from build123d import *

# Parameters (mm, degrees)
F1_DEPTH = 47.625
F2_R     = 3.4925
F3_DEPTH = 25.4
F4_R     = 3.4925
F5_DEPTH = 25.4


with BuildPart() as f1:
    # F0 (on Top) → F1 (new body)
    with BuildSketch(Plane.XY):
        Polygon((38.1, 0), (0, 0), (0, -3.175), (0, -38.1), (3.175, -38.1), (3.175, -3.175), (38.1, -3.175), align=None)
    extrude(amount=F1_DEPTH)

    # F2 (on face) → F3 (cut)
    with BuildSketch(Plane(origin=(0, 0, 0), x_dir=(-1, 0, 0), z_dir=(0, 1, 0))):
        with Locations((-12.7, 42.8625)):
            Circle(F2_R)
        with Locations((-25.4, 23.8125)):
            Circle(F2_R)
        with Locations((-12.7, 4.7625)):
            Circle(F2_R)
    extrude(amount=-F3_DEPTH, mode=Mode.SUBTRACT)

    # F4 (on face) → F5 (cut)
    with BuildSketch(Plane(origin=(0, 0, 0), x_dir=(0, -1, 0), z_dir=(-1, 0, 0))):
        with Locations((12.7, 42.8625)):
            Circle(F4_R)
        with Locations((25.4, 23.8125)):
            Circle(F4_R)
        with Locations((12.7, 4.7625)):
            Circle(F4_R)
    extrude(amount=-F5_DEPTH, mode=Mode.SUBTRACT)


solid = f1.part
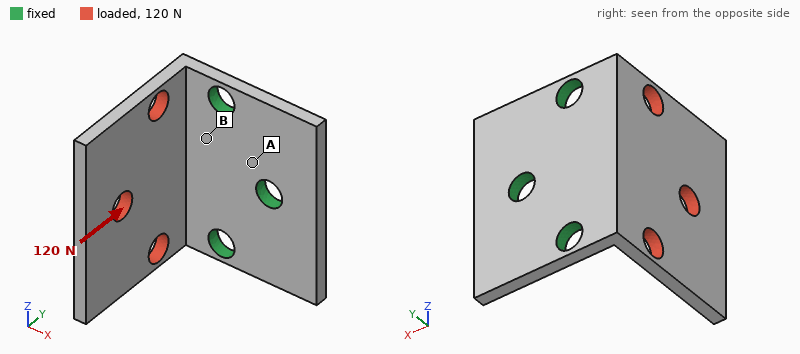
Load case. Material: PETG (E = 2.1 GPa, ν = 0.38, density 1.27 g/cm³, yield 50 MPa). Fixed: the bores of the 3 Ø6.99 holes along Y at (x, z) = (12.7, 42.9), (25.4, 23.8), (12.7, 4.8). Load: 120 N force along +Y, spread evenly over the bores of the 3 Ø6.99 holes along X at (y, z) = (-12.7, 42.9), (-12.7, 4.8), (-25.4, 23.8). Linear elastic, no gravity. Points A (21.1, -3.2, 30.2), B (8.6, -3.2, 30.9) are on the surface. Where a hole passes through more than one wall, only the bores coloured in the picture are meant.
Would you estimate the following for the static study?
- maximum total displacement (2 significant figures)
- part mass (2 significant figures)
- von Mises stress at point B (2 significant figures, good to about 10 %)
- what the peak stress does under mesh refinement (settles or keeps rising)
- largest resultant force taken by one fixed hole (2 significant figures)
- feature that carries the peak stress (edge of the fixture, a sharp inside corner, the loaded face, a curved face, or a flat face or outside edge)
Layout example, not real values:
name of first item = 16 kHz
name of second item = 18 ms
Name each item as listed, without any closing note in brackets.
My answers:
maximum total displacement = 0.71 mm
part mass = 13 g
von Mises stress at point B = 4.3 MPa
what the peak stress does under mesh refinement = keeps rising
largest resultant force taken by one fixed hole = 65 N
feature that carries the peak stress = edge of the fixture
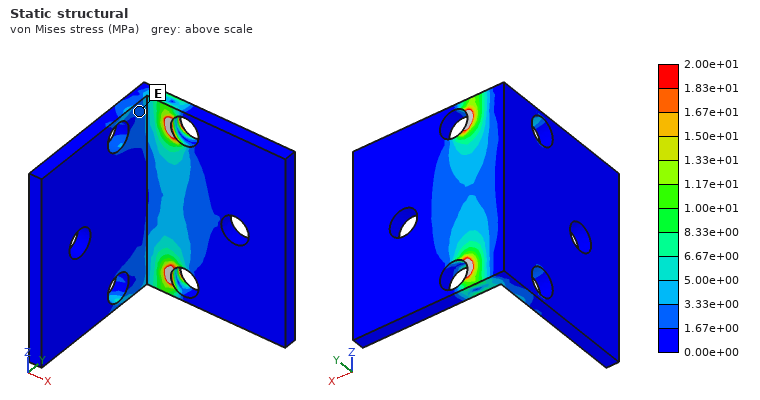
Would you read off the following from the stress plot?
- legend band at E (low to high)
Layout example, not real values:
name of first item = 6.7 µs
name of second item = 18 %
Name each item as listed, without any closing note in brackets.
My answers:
legend band at E = 1.67e+00 to 3.33e+00 MPa
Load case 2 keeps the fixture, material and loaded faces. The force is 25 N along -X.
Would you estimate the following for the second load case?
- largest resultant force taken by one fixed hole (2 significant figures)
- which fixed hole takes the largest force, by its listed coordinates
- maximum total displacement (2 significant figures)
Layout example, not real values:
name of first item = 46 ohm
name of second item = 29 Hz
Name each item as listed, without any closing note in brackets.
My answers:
largest resultant force taken by one fixed hole = 12 N
which fixed hole takes the largest force, by its listed coordinates = (25.4, 23.8)
maximum total displacement = 0.78 mm
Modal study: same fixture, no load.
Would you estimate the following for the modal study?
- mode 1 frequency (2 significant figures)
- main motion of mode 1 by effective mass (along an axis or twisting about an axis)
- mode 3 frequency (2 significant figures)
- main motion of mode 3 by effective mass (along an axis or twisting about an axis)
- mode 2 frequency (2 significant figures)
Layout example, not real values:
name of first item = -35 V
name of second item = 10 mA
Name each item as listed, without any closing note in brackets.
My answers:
mode 1 frequency = 360 Hz
main motion of mode 1 by effective mass = along X
mode 3 frequency = 1500 Hz
main motion of mode 3 by effective mass = along Z
mode 2 frequency = 800 Hz
